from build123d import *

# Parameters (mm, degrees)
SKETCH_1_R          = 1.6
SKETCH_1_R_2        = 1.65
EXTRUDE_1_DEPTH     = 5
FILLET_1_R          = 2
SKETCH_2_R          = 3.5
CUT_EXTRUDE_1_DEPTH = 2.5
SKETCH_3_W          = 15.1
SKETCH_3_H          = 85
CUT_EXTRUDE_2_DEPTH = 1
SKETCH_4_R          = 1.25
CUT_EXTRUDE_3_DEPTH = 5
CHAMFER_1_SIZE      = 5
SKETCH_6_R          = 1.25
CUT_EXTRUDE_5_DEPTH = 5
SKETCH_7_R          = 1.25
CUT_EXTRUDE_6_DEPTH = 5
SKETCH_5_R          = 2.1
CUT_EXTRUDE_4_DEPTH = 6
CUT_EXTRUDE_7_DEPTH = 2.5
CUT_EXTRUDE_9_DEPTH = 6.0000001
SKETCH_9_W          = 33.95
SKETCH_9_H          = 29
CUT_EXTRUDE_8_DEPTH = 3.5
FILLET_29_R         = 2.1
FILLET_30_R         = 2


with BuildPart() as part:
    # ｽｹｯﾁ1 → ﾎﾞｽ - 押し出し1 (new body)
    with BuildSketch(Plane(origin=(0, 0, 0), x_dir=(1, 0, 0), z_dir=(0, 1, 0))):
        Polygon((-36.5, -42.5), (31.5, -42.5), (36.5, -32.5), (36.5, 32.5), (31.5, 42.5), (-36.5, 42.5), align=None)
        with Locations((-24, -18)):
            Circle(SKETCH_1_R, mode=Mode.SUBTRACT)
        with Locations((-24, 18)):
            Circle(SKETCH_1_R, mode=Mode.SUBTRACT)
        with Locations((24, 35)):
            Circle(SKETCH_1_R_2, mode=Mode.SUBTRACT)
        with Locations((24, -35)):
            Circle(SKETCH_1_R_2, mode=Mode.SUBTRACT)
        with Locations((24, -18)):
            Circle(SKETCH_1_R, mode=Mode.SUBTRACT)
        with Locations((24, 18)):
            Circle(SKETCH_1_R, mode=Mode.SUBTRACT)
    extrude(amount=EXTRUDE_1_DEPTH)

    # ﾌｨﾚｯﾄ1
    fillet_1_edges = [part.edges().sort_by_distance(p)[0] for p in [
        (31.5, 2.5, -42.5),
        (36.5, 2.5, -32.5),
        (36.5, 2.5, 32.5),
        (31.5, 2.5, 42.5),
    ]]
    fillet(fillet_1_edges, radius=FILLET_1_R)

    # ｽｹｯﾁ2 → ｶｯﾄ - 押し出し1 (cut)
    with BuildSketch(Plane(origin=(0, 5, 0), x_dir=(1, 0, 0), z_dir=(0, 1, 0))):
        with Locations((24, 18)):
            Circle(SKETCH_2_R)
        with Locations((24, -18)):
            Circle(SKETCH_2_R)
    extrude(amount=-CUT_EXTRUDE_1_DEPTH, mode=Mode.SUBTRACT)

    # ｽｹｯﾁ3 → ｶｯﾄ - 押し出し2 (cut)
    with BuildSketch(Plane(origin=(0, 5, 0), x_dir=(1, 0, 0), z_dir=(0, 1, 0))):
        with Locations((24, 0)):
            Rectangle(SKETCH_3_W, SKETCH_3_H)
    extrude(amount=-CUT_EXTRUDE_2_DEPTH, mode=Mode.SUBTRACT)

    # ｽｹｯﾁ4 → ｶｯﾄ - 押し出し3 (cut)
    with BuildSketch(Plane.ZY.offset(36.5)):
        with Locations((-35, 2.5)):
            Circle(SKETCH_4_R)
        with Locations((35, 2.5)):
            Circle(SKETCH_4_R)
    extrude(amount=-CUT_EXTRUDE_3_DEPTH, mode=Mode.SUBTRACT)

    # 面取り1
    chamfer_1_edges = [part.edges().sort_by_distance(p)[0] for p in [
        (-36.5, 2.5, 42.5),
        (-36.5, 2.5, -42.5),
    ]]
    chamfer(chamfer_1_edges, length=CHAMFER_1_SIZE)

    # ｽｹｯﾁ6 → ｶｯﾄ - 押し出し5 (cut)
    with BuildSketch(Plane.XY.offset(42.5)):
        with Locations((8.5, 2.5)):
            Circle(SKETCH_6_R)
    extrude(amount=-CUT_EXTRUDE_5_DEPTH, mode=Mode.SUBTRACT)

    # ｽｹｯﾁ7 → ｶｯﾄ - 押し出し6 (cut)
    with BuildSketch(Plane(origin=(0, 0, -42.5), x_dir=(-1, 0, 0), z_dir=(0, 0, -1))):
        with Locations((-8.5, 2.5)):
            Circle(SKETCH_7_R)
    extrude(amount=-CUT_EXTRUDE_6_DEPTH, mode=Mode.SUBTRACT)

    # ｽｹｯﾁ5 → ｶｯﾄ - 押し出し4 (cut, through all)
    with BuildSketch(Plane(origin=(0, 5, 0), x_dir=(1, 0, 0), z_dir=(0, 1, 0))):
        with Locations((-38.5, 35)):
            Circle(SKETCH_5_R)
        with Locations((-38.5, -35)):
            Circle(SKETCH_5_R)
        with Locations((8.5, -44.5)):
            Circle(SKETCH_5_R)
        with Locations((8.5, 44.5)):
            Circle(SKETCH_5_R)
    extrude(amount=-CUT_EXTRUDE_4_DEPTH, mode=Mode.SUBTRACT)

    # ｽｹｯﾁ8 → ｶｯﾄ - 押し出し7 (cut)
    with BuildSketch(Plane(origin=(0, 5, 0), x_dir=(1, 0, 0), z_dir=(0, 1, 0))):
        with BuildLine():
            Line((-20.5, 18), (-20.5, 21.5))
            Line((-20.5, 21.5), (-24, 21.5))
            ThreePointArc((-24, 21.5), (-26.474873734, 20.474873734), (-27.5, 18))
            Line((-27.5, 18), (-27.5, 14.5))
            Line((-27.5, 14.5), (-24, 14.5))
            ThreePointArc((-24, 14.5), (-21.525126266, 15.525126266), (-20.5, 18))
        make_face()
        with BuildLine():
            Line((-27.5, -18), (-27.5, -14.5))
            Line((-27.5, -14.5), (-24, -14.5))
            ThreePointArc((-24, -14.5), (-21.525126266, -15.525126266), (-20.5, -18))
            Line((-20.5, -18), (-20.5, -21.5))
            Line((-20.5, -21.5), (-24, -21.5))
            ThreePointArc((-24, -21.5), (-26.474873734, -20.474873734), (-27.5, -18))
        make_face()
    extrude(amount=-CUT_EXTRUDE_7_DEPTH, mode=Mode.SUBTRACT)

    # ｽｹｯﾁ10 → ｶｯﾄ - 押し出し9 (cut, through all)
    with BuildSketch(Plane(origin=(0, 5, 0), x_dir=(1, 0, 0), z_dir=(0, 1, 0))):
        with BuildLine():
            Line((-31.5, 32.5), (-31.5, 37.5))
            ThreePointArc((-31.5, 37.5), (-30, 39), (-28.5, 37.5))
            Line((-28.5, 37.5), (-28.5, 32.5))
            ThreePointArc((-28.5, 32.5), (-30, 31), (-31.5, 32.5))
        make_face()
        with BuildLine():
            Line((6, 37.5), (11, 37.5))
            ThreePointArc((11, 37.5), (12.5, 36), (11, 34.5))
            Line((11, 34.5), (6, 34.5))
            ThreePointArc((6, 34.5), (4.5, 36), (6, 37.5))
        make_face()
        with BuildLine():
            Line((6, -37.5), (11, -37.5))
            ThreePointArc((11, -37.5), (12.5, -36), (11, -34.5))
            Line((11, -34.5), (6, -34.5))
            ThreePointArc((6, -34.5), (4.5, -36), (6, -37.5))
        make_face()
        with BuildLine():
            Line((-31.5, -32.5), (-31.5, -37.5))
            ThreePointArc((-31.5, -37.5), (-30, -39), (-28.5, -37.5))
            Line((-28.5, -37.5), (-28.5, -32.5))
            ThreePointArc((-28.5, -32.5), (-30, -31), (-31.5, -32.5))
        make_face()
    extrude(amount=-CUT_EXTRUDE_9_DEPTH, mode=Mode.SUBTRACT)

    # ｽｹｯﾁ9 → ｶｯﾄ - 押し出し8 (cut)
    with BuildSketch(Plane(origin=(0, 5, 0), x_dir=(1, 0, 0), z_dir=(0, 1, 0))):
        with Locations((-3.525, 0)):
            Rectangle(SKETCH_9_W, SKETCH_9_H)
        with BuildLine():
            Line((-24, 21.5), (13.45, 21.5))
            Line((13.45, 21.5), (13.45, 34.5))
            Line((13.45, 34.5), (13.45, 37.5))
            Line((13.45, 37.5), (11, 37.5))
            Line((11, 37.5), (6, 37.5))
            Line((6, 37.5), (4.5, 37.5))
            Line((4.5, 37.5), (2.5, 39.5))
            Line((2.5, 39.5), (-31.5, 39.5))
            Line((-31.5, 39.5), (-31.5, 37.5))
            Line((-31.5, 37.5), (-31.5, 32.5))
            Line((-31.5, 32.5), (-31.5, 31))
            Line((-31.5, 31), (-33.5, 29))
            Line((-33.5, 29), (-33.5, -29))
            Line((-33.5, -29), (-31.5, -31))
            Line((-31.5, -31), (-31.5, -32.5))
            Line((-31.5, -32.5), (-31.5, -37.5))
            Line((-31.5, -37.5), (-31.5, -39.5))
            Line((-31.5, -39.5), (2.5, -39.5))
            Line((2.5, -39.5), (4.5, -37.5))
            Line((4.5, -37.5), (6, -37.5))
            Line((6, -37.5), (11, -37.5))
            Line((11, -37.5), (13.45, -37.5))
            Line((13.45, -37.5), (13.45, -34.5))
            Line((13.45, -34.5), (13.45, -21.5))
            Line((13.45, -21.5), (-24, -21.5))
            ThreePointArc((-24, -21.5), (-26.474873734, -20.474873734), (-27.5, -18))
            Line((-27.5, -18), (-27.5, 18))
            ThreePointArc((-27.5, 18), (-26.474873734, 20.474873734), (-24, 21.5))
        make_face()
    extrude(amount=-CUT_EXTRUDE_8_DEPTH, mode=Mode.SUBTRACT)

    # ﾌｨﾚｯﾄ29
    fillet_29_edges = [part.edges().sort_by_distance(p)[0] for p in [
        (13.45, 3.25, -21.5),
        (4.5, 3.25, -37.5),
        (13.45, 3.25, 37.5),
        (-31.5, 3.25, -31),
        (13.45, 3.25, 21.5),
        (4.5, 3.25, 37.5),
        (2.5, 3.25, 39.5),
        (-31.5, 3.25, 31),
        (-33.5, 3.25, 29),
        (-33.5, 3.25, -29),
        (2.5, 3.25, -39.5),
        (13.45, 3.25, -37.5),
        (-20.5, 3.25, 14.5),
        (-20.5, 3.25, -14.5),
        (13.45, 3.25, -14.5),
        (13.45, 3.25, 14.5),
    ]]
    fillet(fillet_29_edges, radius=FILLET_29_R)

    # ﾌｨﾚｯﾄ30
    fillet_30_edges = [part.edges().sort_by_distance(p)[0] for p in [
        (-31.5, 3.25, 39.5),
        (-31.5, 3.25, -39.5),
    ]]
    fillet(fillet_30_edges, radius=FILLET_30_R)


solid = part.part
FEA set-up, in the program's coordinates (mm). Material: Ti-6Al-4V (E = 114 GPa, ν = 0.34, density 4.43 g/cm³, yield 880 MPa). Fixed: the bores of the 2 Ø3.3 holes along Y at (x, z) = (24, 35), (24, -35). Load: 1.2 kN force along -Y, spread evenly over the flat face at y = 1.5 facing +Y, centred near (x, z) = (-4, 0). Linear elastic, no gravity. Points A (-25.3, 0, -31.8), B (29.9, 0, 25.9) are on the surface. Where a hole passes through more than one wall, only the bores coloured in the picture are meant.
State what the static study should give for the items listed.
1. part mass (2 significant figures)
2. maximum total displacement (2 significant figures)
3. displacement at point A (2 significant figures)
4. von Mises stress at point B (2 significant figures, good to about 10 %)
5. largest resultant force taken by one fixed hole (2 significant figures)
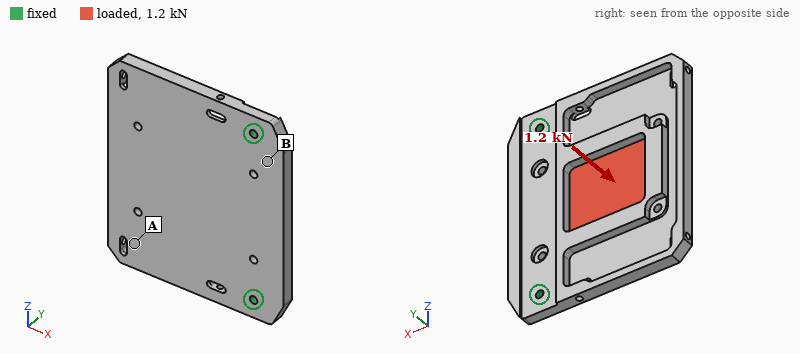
83 g
1.1 mm
0.73 mm
95 MPa
610 N
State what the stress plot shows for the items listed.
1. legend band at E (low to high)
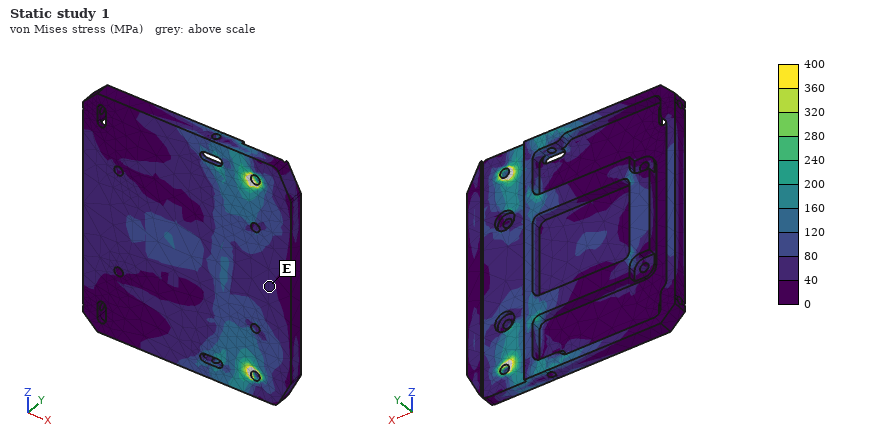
40 to 80 MPa
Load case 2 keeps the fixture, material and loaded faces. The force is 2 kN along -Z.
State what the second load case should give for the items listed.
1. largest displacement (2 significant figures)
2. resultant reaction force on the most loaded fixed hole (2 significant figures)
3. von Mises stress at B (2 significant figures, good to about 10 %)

26 µm
1.3 kN
6.2 MPa
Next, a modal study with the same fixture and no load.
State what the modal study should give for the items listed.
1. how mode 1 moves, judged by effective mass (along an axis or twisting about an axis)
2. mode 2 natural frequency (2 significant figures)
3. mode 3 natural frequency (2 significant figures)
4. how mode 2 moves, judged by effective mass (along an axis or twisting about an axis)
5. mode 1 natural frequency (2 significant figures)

along Y
1500 Hz
3300 Hz
twisting about X
810 Hz
